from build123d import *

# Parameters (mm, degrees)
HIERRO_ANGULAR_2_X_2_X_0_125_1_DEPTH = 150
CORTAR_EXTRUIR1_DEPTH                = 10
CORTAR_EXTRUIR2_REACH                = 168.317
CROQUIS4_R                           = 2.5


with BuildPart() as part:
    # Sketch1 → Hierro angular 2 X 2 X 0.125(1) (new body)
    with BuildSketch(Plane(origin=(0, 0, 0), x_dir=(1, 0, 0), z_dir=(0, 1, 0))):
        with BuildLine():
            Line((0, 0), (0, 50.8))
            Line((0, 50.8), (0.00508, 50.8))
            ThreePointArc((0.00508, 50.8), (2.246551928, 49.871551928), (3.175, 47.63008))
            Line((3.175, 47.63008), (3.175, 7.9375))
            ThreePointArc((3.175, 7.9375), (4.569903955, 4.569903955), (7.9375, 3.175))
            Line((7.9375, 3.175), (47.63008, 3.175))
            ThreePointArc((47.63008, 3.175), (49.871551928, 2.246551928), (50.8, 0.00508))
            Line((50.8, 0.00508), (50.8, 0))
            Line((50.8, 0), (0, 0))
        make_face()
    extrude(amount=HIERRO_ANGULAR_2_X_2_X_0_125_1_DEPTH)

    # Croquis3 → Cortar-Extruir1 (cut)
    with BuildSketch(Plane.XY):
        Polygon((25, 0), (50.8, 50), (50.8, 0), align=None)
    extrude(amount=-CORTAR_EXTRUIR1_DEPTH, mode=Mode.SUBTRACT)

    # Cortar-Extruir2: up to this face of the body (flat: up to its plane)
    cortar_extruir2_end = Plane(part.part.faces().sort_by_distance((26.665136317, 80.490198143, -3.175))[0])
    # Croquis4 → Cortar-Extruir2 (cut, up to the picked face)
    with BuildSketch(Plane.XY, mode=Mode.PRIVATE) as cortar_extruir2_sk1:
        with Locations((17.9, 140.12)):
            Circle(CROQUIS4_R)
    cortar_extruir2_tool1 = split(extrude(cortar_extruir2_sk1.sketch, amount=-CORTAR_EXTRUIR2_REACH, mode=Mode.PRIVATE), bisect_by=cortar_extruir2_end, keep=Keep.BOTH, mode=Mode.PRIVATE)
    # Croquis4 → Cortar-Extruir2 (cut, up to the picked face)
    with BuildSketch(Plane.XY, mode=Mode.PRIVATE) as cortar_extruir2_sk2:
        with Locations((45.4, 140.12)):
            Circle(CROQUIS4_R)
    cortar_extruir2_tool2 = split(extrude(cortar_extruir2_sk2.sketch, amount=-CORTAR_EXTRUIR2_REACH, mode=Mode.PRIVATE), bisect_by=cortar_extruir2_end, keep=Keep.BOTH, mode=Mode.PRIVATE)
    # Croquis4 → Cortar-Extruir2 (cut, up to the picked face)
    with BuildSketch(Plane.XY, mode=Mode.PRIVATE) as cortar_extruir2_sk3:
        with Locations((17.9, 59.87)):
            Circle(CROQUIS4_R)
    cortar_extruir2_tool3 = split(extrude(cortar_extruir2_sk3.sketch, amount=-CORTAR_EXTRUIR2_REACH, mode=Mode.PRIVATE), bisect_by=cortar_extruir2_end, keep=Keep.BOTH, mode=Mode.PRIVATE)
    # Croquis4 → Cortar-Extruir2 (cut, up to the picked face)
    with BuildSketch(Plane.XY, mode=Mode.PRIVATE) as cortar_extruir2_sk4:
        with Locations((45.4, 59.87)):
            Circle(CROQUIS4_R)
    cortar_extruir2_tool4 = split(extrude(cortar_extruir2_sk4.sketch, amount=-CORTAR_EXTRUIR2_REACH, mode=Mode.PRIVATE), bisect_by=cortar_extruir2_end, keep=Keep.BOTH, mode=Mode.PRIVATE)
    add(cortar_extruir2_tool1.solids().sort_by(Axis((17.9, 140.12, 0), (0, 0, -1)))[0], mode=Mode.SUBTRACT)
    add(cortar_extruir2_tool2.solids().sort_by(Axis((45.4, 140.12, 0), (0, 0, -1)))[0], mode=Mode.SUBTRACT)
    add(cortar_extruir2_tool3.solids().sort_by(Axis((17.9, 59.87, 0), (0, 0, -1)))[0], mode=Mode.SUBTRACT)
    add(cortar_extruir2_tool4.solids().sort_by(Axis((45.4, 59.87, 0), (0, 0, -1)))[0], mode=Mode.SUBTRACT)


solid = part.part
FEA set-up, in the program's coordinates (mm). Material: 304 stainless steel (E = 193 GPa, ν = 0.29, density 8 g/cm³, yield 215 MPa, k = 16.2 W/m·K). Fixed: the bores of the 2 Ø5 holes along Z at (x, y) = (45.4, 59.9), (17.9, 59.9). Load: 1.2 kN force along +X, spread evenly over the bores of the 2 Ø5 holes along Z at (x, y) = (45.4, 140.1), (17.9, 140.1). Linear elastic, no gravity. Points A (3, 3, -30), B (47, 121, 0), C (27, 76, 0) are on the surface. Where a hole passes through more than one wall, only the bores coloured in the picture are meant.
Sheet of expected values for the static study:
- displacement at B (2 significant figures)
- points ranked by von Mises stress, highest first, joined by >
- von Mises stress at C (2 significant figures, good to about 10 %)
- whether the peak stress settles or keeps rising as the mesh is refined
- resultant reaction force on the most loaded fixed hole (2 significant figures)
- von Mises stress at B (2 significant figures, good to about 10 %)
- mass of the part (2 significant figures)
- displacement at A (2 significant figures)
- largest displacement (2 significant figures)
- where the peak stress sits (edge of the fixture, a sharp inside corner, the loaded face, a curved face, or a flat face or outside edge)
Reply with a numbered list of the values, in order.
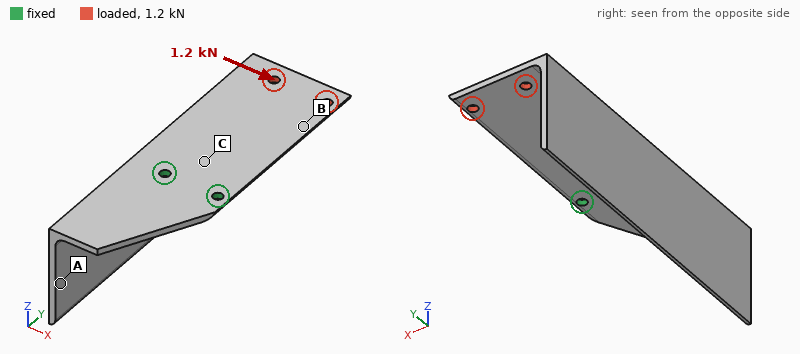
1. 36 µm
2. C > B > A
3. 26 MPa
4. keeps rising
5. 3.3 kN
6. 13 MPa
7. 360 g
8. 15 µm
9. 58 µm
10. edge of the fixture
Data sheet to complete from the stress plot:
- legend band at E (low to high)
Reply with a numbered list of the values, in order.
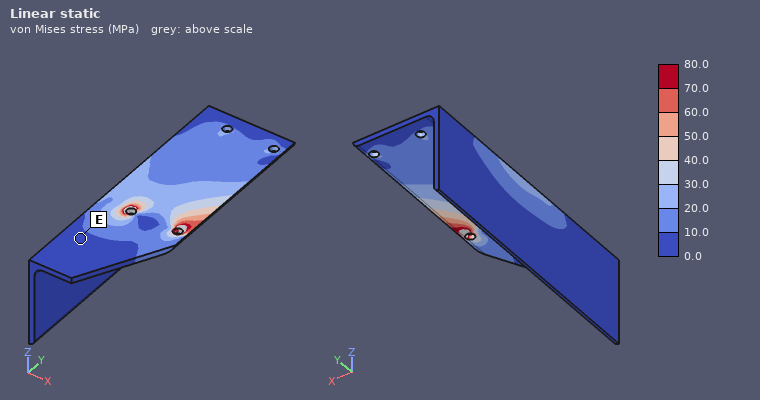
1. 0.0 to 10.0 MPa
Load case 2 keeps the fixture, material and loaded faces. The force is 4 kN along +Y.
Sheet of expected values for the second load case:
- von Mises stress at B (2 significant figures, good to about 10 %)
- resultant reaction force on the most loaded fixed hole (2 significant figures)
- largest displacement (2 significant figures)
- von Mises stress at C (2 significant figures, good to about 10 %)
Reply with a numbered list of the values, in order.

1. 44 MPa
2. 2.0 kN
3. 28 µm
4. 24 MPa
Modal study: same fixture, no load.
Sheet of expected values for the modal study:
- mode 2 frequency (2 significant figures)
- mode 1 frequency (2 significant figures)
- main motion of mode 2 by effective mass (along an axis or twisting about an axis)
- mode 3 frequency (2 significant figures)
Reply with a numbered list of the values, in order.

1. 540 Hz
2. 330 Hz
3. along X
4. 870 Hz
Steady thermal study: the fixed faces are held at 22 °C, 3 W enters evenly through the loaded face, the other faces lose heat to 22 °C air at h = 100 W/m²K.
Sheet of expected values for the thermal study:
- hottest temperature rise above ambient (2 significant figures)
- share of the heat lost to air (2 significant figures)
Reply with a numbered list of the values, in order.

1. 20 K
2. 100 %
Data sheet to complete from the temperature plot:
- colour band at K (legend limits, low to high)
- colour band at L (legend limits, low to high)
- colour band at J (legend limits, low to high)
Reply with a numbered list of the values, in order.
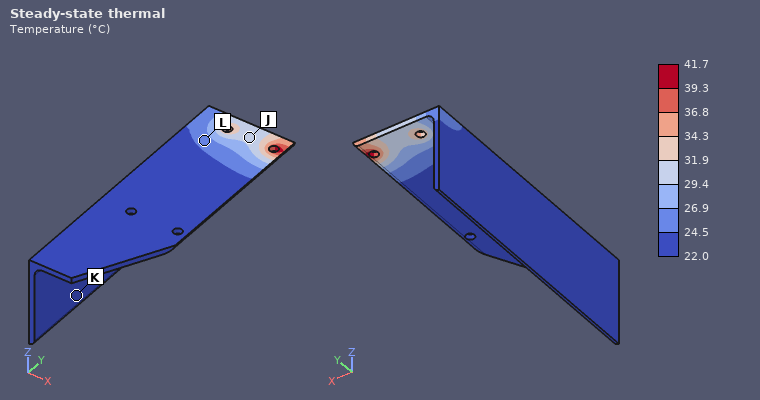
1. 22.0 to 24.5 °C
2. 24.5 to 26.9 °C
3. 29.4 to 31.9 °C
